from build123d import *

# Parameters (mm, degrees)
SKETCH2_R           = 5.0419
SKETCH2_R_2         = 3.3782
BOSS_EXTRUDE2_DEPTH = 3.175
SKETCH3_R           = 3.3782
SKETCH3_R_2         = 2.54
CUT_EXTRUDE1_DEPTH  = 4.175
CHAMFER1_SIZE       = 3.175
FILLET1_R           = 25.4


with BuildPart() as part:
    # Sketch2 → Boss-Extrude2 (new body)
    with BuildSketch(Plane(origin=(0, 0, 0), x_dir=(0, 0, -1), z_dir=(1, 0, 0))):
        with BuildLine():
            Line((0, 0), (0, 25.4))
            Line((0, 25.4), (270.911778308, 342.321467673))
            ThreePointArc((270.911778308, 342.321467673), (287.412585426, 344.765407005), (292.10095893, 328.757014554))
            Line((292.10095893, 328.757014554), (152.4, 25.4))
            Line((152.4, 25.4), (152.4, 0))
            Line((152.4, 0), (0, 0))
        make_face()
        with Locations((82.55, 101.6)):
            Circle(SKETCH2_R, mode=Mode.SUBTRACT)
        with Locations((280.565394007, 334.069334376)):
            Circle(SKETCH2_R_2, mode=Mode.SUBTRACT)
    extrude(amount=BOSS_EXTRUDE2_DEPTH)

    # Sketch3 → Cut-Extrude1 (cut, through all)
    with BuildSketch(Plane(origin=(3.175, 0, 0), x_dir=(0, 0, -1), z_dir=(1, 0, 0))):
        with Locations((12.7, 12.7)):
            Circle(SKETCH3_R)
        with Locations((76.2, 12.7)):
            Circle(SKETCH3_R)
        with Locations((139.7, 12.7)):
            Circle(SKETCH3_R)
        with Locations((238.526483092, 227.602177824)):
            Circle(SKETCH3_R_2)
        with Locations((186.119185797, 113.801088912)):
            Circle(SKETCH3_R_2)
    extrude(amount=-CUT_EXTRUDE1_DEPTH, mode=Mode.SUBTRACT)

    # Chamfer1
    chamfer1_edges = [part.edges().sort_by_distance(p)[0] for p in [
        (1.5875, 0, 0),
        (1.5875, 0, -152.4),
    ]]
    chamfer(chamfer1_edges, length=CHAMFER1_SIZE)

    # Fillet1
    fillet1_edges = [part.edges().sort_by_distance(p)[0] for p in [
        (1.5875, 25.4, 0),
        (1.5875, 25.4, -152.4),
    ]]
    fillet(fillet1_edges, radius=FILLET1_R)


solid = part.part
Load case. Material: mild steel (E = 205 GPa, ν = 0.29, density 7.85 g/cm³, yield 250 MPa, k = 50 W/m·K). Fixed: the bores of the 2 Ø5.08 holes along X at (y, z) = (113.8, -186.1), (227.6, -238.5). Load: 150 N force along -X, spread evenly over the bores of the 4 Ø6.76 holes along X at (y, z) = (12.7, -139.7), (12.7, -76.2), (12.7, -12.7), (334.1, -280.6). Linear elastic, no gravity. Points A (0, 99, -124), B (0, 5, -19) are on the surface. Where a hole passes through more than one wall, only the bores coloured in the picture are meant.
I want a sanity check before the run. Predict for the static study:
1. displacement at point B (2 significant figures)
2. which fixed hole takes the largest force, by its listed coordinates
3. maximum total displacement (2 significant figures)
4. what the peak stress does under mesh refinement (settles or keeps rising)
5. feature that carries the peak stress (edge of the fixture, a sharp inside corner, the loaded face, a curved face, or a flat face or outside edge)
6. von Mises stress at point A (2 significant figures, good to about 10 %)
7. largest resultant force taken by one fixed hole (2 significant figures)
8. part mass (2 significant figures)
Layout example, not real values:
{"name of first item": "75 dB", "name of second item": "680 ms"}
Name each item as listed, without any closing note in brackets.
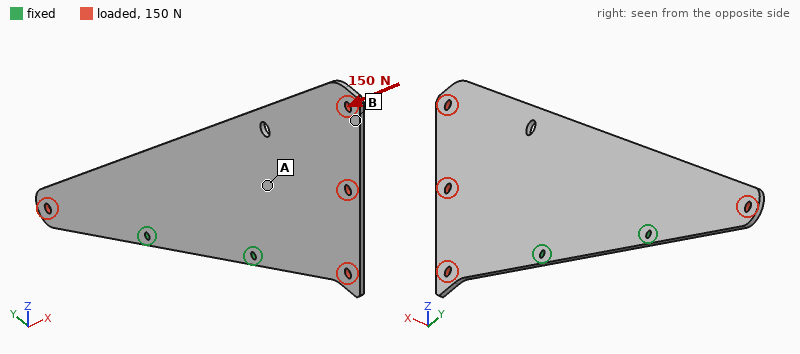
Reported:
{"displacement at point B": "4.2 mm", "which fixed hole takes the largest force, by its listed coordinates": "(113.8, -186.1)", "maximum total displacement": "4.6 mm", "what the peak stress does under mesh refinement": "keeps rising", "feature that carries the peak stress": "edge of the fixture", "von Mises stress at point A": "60 MPa", "largest resultant force taken by one fixed hole": "170 N", "part mass": "800 g"}
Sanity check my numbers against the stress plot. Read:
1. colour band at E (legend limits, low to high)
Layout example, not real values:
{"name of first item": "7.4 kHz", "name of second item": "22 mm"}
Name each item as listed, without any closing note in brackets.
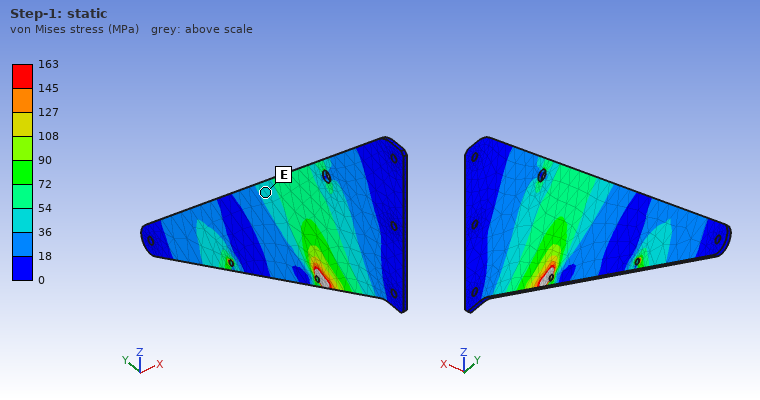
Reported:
{"colour band at E": "36 to 54 MPa"}
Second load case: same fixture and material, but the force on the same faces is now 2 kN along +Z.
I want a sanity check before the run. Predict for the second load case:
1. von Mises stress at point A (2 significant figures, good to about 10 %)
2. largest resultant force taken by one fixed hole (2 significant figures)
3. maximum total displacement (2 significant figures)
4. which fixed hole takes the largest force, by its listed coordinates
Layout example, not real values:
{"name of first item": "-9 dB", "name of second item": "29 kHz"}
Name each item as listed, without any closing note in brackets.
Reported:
{"von Mises stress at point A": "12 MPa", "largest resultant force taken by one fixed hole": "3.2 kN", "maximum total displacement": "85 µm", "which fixed hole takes the largest force, by its listed coordinates": "(113.8, -186.1)"}
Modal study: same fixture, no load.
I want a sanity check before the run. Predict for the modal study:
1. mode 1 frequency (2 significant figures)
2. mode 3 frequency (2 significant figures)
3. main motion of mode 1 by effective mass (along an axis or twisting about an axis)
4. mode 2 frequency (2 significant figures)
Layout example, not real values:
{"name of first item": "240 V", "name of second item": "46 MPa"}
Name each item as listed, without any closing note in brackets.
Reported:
{"mode 1 frequency": "68 Hz", "mode 3 frequency": "220 Hz", "main motion of mode 1 by effective mass": "along X", "mode 2 frequency": "200 Hz"}
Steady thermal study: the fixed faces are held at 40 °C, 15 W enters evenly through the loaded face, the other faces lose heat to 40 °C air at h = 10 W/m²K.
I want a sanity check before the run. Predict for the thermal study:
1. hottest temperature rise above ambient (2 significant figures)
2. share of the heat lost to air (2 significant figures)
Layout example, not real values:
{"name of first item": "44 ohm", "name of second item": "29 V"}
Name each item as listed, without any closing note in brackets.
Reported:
{"hottest temperature rise above ambient": "54 K", "share of the heat lost to air": "78 %"}
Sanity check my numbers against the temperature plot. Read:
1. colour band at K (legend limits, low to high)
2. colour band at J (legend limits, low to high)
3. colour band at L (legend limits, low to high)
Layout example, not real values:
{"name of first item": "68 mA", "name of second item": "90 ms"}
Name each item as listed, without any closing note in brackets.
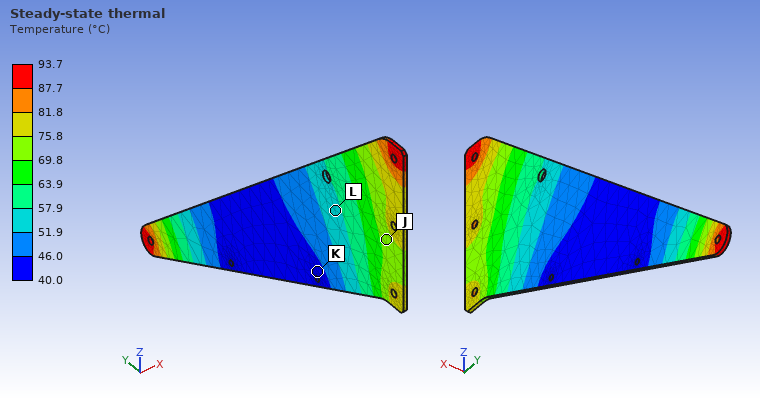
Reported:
{"colour band at K": "40.0 to 46.0 °C", "colour band at J": "69.8 to 75.8 °C", "colour band at L": "51.9 to 57.9 °C"}
